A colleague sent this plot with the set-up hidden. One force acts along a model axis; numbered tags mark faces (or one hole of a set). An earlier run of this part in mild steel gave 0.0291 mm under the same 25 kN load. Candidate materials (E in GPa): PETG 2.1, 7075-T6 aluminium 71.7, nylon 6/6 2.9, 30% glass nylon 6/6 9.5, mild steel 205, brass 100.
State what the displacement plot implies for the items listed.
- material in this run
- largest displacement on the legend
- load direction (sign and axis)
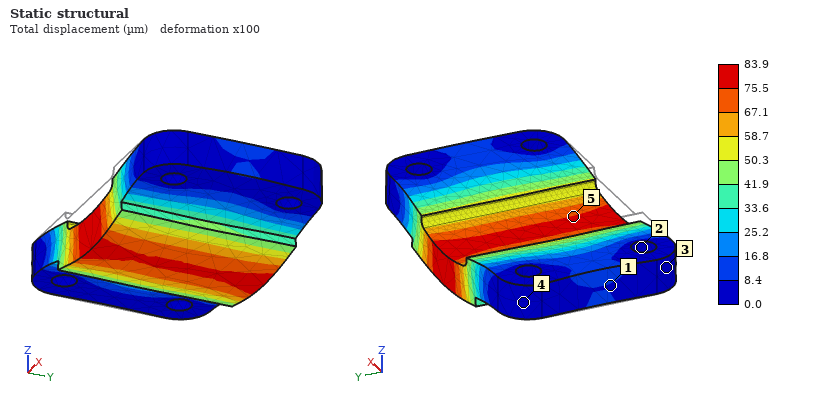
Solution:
7075-T6 aluminium
83.9 µm
-Z
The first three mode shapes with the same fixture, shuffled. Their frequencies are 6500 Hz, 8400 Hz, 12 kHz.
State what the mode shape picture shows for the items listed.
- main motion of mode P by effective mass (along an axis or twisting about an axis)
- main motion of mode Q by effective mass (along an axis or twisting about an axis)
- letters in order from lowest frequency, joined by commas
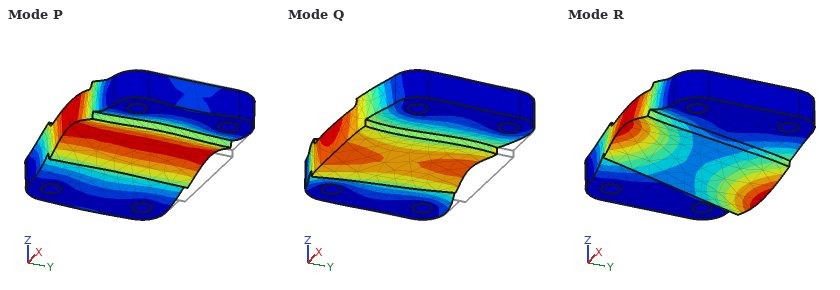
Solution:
along Z
along Y
P, R, Q
